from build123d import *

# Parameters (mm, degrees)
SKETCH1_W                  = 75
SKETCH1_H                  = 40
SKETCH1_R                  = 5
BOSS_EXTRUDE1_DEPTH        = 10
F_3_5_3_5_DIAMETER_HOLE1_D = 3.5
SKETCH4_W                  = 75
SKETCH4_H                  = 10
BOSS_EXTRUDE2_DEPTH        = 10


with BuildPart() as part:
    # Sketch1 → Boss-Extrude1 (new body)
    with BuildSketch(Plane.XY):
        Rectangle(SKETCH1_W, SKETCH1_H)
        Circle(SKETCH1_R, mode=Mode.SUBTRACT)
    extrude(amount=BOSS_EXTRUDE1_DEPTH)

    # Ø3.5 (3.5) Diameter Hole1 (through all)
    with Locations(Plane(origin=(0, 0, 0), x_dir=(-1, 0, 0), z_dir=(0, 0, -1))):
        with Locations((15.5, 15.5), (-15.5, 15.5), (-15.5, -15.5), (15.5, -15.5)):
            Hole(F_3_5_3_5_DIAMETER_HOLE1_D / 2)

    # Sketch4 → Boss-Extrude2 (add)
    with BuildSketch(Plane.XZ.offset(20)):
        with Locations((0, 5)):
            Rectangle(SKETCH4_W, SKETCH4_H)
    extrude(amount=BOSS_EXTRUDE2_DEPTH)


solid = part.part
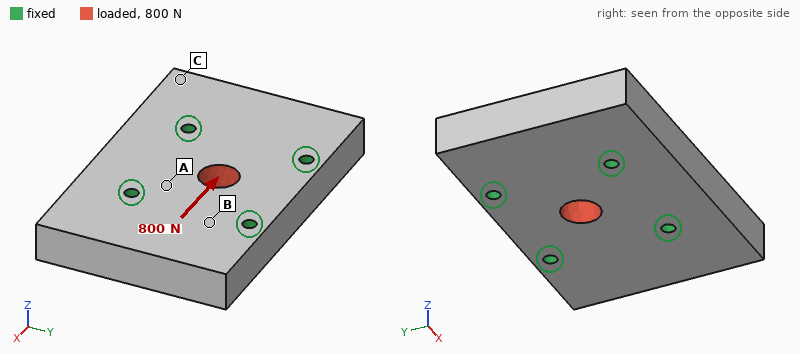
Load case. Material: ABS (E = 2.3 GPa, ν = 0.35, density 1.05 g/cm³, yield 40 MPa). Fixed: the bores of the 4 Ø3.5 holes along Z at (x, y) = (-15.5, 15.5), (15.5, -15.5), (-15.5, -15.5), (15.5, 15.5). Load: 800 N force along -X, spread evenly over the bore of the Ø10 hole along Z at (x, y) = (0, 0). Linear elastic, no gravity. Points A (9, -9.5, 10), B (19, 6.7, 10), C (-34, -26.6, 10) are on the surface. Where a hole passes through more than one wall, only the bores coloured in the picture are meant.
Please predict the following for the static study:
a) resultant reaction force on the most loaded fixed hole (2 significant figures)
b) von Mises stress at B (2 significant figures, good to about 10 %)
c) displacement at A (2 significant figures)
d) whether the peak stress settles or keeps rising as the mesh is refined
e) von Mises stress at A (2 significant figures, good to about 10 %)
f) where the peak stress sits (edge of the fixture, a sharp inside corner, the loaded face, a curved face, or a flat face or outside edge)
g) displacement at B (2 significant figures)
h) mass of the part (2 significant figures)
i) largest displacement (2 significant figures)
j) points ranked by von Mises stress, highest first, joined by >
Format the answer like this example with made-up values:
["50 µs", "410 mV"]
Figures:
["210 N", "0.85 MPa", "7.2 µm", "keeps rising", "1.7 MPa", "edge of the fixture", "7.3 µm", "38 g", "18 µm", "A > B > C"]
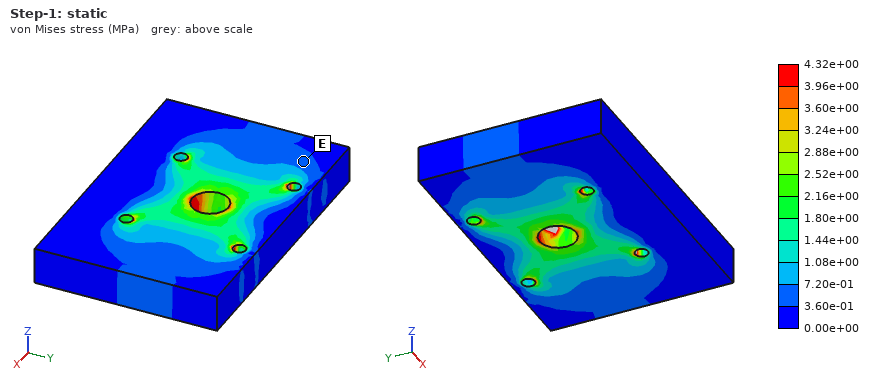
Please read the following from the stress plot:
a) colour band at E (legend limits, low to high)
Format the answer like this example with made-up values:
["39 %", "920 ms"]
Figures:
["3.60e-01 to 7.20e-01 MPa"]
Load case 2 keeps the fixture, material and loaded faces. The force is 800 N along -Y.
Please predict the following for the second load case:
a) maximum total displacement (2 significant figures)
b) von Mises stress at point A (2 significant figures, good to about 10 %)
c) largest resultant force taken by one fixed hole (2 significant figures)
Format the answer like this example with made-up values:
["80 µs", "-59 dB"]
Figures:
["23 µm", "1.9 MPa", "230 N"]
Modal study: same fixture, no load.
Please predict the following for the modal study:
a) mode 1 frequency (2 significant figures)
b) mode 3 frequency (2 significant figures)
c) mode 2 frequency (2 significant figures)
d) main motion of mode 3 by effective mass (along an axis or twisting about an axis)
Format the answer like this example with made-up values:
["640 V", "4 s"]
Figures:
["3500 Hz", "4800 Hz", "3600 Hz", "twisting about X"]
